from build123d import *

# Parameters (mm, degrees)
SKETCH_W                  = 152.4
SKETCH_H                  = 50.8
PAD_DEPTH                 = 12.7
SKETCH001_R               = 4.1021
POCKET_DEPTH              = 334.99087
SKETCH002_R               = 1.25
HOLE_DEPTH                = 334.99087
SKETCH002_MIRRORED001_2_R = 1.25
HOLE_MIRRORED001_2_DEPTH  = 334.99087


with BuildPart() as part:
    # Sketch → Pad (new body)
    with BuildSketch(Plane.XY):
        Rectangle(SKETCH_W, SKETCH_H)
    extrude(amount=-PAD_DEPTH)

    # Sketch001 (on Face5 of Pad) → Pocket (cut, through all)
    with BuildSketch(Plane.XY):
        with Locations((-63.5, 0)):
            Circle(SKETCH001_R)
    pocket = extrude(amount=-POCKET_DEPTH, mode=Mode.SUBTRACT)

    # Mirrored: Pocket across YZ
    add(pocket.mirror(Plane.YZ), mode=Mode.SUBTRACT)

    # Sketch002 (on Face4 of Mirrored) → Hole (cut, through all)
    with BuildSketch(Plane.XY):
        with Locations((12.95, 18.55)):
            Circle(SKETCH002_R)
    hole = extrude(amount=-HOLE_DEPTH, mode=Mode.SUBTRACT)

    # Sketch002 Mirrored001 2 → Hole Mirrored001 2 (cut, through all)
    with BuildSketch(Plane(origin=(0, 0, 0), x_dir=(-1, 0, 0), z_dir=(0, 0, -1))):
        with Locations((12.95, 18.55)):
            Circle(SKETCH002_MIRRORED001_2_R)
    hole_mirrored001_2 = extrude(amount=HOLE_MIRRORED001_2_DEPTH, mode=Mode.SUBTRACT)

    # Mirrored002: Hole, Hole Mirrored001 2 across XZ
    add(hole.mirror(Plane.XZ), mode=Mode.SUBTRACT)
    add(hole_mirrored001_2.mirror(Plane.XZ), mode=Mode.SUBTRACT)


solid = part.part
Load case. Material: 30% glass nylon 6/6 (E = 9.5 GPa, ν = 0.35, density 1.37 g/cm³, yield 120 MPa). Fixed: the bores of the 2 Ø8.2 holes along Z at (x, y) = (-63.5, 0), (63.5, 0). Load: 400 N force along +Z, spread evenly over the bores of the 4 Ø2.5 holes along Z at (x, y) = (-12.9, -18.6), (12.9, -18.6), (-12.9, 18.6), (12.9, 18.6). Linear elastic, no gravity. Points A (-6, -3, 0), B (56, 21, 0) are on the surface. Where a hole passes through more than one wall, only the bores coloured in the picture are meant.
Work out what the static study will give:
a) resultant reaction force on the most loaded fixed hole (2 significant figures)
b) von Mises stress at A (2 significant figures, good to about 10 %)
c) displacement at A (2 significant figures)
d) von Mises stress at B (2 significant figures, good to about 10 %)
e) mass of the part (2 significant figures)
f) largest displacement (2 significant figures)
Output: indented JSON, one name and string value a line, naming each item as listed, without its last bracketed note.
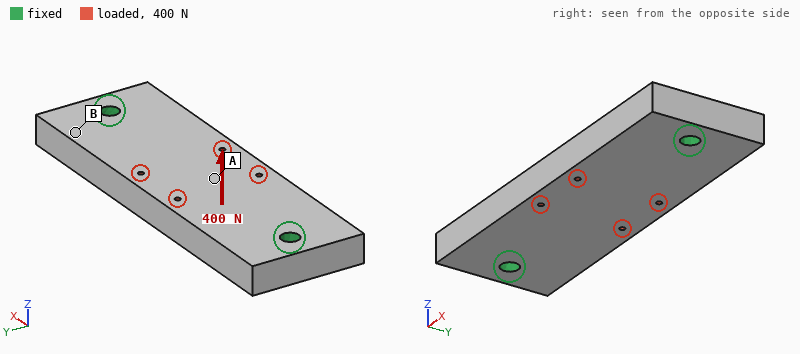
{
  "resultant reaction force on the most loaded fixed hole": "200 N",
  "von Mises stress at A": "3.2 MPa",
  "displacement at A": "56 µm",
  "von Mises stress at B": "1.8 MPa",
  "mass of the part": "130 g",
  "largest displacement": "64 µm"
}
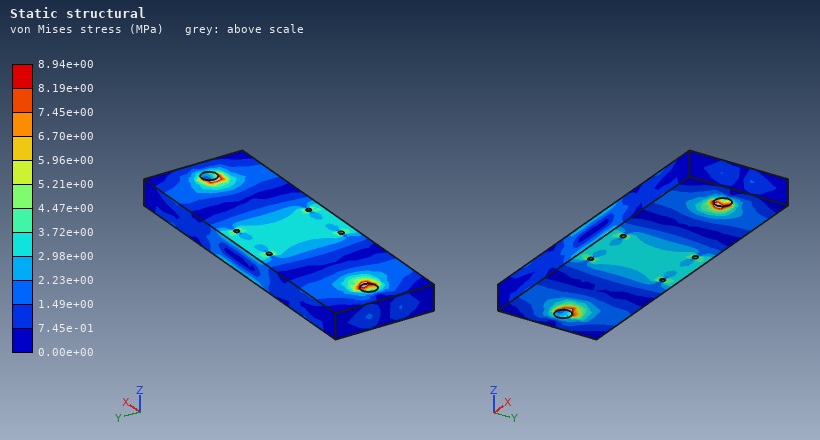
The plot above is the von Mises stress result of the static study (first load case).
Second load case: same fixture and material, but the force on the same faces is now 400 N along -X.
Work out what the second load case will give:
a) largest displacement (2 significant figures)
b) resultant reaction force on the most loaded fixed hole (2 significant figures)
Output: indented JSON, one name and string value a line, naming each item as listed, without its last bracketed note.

{
  "largest displacement": "2.7 µm",
  "resultant reaction force on the most loaded fixed hole": "200 N"
}
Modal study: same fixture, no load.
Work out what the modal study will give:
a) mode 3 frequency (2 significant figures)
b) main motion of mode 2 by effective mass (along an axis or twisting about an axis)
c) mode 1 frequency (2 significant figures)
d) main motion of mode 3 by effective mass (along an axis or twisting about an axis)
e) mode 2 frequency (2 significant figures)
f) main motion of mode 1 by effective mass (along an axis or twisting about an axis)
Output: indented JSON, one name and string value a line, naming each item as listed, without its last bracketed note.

{
  "mode 3 frequency": "3400 Hz",
  "main motion of mode 2 by effective mass": "twisting about X",
  "mode 1 frequency": "1800 Hz",
  "main motion of mode 3 by effective mass": "along Y",
  "mode 2 frequency": "2700 Hz",
  "main motion of mode 1 by effective mass": "along Z"
}
